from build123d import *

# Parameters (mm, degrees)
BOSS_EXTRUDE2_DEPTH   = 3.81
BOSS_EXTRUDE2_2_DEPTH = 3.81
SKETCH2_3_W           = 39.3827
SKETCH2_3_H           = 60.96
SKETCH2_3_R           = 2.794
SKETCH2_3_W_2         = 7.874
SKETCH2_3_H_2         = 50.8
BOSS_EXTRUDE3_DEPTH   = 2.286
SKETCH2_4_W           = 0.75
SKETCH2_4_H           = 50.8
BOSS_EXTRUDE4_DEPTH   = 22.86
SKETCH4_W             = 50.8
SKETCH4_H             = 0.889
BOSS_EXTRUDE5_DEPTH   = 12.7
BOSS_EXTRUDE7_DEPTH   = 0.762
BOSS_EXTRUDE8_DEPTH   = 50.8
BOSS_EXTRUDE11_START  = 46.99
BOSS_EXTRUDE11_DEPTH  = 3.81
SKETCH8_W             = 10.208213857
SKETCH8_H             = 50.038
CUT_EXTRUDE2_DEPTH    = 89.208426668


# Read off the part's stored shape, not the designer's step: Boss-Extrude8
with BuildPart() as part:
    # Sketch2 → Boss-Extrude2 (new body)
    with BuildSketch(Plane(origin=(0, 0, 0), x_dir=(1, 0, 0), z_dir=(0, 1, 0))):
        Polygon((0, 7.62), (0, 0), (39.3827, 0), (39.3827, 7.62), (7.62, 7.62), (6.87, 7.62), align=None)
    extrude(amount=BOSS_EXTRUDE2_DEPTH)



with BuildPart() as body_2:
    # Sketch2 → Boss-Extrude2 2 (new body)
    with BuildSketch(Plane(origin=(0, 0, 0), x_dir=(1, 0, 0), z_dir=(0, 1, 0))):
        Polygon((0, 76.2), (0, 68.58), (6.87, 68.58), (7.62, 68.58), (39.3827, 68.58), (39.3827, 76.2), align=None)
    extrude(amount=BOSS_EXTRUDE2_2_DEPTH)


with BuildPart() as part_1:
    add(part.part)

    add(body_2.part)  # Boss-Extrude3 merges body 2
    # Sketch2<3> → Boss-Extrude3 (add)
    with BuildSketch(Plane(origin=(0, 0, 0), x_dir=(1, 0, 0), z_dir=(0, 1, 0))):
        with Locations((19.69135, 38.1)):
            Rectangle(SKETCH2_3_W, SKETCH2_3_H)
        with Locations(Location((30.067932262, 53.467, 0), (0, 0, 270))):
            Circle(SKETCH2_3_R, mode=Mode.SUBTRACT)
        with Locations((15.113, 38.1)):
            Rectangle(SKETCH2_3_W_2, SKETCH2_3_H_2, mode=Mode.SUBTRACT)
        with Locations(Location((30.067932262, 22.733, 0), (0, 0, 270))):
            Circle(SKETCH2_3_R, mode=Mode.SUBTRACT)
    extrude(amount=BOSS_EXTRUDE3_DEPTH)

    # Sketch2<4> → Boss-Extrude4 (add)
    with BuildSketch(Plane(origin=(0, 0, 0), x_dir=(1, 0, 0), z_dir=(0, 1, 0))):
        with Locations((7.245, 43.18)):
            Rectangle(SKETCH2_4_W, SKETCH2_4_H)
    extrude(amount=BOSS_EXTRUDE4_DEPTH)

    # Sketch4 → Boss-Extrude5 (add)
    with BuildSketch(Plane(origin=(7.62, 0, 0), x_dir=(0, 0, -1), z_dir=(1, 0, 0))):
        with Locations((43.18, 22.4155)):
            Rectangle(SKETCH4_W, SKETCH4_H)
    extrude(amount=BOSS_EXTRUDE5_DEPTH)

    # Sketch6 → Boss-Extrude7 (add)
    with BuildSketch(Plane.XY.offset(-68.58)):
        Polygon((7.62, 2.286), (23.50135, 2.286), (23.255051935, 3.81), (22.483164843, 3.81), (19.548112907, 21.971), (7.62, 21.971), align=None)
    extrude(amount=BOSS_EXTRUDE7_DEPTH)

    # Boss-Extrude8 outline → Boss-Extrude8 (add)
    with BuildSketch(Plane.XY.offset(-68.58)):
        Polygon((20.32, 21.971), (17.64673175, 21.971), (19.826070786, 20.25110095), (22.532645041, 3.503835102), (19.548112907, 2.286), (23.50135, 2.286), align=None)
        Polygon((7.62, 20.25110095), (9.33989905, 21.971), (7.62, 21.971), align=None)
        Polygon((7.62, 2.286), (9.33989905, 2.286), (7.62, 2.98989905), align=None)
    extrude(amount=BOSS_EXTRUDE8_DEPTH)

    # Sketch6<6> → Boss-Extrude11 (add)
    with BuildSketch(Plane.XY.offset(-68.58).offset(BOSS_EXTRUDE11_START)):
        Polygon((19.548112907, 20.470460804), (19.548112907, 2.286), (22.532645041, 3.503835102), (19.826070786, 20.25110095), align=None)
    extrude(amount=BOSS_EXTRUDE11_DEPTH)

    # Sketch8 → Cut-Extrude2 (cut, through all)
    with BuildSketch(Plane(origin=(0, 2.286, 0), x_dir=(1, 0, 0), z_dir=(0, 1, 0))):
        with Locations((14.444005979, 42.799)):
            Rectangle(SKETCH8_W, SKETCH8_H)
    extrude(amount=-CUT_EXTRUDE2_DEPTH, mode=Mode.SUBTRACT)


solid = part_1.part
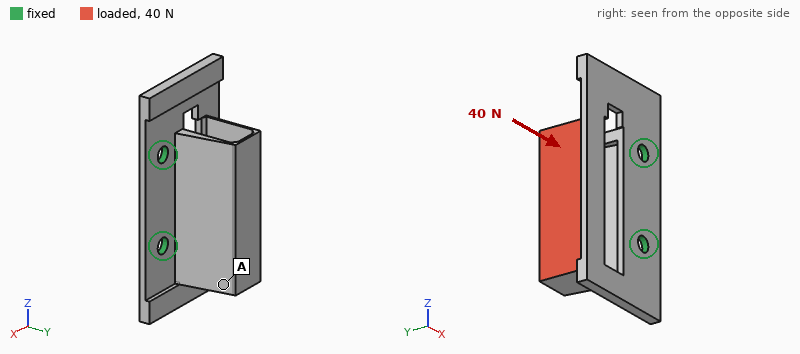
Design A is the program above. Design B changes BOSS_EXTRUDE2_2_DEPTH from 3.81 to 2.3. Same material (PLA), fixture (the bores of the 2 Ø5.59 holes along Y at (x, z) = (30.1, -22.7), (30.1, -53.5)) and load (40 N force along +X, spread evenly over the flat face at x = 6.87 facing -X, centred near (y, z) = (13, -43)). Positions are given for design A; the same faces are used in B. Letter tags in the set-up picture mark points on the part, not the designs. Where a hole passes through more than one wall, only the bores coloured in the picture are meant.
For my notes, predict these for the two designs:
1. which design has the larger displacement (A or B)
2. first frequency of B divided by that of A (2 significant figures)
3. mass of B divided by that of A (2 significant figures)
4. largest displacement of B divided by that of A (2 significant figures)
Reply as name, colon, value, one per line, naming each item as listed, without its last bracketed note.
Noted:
which design has the larger displacement: B
first frequency of B divided by that of A: 0.94
mass of B divided by that of A: 0.95
largest displacement of B divided by that of A: 1.1
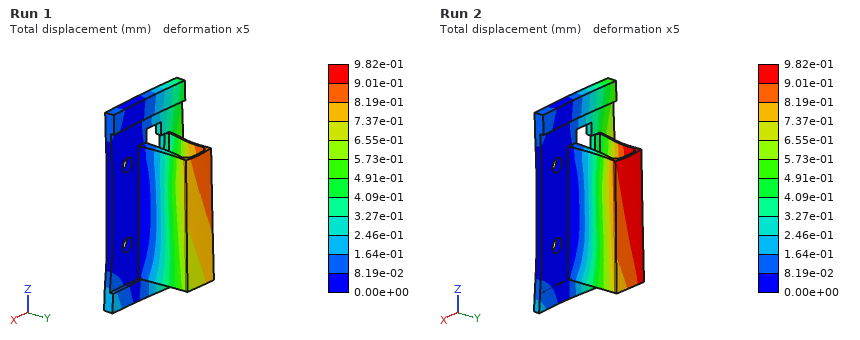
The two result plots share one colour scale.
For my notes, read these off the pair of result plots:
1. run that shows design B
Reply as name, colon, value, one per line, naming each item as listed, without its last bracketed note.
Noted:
run that shows design B: Run 2
